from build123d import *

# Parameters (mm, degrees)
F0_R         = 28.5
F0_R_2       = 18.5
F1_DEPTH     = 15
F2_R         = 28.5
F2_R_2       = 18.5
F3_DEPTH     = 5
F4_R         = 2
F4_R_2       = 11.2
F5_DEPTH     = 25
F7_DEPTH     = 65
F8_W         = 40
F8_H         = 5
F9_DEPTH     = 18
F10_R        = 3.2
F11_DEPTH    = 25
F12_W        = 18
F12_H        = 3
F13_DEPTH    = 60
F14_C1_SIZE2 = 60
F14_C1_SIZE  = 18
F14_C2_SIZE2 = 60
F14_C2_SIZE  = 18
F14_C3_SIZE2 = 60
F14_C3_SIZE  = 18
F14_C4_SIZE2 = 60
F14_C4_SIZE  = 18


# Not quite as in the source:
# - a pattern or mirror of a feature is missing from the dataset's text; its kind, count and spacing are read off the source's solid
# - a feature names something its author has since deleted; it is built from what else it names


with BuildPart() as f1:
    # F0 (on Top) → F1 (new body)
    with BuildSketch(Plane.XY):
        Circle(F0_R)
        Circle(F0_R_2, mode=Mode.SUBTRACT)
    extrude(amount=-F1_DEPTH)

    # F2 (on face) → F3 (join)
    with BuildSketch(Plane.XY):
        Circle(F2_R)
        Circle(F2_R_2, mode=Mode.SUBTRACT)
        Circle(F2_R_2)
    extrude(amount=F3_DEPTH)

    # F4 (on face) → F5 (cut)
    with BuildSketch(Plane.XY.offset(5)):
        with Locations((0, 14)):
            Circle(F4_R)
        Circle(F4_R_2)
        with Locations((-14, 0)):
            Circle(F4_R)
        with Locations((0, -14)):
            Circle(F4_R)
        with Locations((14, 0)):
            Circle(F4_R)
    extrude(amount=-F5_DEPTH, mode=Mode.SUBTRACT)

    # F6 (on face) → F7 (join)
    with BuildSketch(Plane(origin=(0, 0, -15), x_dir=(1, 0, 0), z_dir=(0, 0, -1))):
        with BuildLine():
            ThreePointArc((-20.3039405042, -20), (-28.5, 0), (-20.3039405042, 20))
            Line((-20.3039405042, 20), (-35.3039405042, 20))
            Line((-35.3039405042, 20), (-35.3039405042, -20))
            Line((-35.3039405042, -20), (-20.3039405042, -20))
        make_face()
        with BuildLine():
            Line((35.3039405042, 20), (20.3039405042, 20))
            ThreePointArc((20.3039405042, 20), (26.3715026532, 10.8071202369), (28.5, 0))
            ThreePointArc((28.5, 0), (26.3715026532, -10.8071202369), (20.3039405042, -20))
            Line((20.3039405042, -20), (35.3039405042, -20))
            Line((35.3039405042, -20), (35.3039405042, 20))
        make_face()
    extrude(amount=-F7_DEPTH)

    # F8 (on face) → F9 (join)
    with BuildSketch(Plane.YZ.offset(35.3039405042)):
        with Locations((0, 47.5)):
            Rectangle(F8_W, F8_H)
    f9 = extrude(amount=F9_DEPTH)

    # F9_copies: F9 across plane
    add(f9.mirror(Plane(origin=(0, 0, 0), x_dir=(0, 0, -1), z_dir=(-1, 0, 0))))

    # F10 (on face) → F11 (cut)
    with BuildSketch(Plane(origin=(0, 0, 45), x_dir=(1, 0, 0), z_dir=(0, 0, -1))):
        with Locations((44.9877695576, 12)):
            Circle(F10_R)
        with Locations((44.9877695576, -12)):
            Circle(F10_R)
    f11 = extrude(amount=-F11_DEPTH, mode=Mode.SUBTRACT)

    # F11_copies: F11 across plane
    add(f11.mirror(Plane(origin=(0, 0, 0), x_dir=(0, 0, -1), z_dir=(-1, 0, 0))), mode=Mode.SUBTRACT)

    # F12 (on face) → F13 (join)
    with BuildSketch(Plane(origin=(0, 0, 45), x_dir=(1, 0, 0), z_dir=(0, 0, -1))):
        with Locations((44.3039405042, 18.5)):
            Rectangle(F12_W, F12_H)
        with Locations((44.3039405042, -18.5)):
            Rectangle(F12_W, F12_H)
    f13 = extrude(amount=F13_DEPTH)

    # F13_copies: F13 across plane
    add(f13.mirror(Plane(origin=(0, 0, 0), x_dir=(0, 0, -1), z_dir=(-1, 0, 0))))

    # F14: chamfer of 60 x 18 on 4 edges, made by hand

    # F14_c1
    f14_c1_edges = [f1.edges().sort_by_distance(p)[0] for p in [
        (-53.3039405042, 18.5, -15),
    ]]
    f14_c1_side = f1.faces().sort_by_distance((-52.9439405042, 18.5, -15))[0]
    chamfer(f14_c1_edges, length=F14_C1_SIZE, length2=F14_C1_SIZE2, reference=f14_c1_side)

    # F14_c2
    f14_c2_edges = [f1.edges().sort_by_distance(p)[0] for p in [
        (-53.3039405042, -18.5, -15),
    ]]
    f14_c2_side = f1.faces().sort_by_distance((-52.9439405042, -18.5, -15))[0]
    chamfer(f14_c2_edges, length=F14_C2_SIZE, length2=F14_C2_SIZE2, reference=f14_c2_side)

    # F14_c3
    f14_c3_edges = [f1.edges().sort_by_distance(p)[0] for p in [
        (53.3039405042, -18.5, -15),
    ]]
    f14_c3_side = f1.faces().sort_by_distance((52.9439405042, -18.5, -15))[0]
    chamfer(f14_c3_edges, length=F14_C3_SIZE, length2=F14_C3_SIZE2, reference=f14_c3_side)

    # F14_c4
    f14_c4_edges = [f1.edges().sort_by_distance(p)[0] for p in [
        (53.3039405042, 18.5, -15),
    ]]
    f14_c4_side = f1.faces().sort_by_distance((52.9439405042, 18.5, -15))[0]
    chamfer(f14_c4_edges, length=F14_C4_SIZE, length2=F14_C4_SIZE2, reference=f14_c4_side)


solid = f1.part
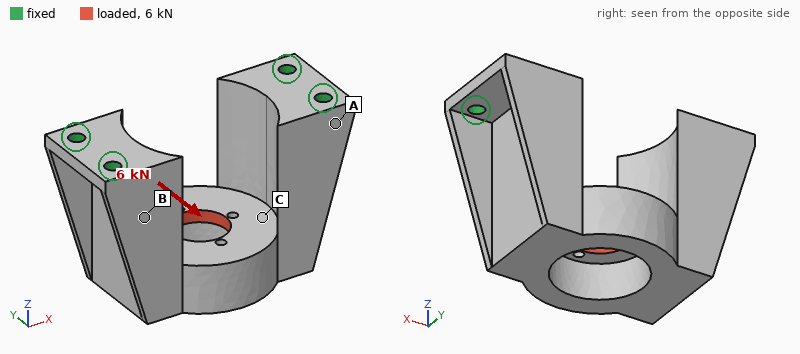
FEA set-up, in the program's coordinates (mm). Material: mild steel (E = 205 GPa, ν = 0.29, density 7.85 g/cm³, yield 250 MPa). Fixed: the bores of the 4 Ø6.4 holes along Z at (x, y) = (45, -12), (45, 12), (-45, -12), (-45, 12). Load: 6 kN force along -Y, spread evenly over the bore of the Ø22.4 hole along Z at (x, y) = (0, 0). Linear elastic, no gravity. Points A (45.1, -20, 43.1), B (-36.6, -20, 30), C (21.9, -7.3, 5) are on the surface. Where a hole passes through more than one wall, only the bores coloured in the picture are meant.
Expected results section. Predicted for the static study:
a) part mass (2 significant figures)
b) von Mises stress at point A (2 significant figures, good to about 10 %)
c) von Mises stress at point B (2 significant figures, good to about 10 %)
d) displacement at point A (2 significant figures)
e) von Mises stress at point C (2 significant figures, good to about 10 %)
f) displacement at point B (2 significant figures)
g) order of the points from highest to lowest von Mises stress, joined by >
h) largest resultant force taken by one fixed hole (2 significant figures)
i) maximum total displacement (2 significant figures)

740 g
69 MPa
39 MPa
9.1 µm
17 MPa
23 µm
A > B > C
5.1 kN
59 µm
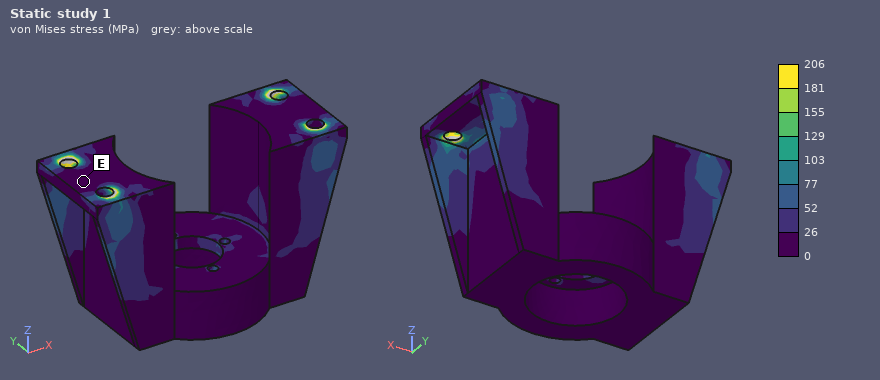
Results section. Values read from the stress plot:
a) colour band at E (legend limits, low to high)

0 to 26 MPa
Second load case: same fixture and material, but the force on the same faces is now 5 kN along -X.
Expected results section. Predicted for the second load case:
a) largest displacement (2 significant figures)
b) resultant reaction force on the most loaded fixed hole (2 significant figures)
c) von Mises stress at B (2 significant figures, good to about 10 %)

38 µm
1.6 kN
34 MPa
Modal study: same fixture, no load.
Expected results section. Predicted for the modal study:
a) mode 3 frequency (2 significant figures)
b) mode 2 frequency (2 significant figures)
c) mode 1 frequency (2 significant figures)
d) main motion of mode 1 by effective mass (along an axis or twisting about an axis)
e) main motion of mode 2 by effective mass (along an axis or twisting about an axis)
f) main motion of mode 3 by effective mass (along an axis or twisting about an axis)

3500 Hz
2700 Hz
2400 Hz
along Y
along X
twisting about Z
